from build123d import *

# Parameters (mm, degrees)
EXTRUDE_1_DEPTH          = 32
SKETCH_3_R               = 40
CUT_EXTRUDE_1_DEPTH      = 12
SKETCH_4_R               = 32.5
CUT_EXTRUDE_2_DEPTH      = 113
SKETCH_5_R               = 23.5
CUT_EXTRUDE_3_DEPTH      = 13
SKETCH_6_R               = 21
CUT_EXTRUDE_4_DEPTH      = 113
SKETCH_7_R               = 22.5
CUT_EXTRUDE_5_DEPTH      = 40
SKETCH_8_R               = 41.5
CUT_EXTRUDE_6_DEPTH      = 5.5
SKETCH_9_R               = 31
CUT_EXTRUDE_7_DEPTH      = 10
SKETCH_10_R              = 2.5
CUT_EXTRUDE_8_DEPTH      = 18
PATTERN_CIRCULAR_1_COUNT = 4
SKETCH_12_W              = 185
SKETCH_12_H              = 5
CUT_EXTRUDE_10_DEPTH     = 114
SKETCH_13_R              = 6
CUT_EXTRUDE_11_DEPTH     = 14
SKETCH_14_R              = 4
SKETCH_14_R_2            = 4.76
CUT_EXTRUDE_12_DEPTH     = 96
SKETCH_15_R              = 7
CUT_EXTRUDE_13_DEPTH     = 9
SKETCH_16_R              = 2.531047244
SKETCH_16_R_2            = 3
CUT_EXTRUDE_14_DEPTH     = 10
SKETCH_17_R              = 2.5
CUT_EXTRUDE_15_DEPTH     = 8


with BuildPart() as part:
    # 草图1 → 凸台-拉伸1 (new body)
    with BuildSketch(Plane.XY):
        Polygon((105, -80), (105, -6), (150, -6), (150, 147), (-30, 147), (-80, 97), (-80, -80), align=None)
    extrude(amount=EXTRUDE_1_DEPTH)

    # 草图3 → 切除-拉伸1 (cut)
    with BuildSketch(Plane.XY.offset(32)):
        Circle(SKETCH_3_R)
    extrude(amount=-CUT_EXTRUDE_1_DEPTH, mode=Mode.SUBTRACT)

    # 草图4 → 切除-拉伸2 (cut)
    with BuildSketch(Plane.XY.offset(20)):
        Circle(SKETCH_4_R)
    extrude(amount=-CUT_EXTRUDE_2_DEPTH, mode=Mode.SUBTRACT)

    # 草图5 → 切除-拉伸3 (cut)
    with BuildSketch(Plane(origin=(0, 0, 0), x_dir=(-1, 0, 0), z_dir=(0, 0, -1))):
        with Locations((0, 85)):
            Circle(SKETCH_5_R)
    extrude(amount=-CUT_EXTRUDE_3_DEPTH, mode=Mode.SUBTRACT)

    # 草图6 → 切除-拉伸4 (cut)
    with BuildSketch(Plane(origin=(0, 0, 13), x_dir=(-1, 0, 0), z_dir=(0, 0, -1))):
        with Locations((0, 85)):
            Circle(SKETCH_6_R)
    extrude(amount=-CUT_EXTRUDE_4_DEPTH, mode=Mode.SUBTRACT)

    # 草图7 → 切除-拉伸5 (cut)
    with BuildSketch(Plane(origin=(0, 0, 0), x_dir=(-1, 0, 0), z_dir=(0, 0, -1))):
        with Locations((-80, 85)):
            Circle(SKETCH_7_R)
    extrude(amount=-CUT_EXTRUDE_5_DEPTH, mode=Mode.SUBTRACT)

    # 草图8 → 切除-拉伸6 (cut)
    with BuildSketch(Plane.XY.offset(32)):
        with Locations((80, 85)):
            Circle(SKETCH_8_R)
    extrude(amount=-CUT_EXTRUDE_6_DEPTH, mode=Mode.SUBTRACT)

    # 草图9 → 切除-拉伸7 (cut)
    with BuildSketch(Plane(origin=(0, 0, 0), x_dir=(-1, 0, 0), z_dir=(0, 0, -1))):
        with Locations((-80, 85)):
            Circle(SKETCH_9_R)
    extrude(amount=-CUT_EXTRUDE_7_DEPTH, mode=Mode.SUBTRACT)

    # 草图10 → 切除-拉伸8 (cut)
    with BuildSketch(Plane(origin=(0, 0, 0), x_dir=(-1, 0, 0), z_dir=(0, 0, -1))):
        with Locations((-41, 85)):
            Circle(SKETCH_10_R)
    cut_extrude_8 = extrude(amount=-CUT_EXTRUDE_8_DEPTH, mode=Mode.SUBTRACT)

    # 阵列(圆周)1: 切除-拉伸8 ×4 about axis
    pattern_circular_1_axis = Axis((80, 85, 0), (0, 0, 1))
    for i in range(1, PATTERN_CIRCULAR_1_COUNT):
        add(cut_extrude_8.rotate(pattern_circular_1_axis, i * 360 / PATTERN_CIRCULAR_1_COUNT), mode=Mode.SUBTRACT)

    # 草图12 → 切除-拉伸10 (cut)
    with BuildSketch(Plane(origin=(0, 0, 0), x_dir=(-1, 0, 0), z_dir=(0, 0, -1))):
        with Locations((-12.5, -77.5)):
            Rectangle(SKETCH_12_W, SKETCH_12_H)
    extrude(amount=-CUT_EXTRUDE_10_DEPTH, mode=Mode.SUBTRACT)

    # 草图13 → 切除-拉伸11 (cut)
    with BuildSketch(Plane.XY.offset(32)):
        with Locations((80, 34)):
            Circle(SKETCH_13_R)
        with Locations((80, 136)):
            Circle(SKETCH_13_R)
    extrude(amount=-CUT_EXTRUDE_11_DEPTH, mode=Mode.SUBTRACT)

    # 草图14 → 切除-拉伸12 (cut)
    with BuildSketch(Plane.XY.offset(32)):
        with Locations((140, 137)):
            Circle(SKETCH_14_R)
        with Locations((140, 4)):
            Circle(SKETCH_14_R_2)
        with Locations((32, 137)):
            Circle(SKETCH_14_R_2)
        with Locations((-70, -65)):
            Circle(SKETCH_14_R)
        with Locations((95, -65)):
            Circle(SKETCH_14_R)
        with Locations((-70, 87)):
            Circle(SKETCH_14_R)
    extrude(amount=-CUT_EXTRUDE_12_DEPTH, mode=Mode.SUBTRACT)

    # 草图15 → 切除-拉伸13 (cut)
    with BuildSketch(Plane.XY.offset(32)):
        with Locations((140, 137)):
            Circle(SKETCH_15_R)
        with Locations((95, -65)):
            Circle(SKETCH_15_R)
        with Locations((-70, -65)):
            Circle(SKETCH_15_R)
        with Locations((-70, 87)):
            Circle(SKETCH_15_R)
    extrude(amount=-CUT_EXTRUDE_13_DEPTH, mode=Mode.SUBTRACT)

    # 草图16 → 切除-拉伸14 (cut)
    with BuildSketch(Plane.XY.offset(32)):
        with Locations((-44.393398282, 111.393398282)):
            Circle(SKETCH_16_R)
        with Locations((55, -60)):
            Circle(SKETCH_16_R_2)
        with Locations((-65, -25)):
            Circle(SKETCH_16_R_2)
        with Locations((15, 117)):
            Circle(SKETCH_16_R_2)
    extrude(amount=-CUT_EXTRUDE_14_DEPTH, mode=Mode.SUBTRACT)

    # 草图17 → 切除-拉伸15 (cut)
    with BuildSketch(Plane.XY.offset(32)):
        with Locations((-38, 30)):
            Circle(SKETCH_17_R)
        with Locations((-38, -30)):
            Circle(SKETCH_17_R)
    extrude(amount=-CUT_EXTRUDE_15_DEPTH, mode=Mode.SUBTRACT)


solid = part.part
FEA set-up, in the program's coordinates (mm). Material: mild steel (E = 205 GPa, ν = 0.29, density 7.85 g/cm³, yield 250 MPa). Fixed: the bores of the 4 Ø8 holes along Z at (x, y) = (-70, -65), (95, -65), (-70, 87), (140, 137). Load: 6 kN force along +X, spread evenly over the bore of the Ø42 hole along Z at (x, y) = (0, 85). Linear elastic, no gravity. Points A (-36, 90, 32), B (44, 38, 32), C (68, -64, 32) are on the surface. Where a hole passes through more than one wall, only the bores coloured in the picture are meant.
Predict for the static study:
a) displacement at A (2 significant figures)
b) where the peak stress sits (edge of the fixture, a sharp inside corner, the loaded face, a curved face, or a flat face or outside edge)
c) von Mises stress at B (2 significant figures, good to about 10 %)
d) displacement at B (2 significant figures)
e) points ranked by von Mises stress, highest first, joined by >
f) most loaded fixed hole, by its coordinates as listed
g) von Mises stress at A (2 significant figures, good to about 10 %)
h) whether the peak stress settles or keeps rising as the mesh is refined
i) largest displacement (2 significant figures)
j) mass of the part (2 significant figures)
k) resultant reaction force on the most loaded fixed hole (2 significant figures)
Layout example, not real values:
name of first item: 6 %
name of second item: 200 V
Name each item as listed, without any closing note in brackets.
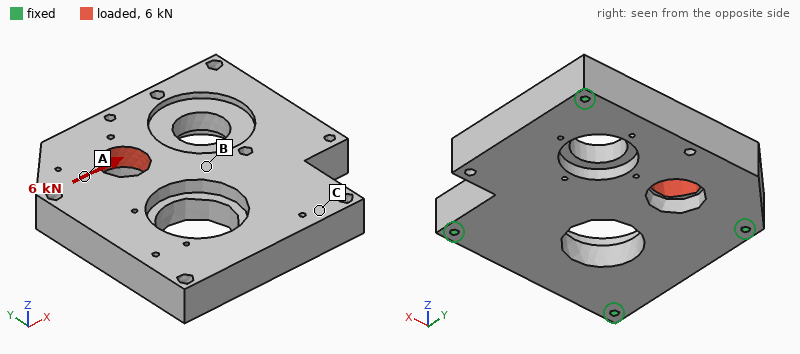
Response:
displacement at A: 0.93 µm
where the peak stress sits: edge of the fixture
von Mises stress at B: 1.1 MPa
displacement at B: 0.99 µm
points ranked by von Mises stress, highest first, joined by >: A > B > C
most loaded fixed hole, by its coordinates as listed: (-70, 87)
von Mises stress at A: 2.9 MPa
whether the peak stress settles or keeps rising as the mesh is refined: keeps rising
largest displacement: 1.6 µm
mass of the part: 9.5 kg
resultant reaction force on the most loaded fixed hole: 3.3 kN
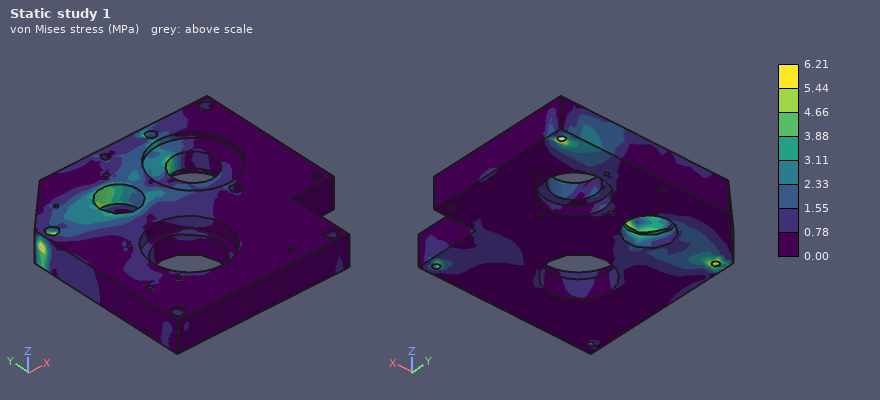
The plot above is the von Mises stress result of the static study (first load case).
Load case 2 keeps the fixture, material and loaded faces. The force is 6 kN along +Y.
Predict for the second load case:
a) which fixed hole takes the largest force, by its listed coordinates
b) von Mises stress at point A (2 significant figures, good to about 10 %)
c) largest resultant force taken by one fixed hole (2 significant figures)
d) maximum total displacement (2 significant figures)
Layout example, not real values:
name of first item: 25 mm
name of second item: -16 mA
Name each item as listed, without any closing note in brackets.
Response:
which fixed hole takes the largest force, by its listed coordinates: (-70, 87)
von Mises stress at point A: 2.0 MPa
largest resultant force taken by one fixed hole: 2.1 kN
maximum total displacement: 2.6 µm
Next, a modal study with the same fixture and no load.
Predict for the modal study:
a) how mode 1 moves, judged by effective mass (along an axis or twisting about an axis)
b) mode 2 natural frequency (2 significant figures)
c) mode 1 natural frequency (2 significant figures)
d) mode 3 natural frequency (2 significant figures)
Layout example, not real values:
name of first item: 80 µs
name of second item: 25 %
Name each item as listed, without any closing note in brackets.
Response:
how mode 1 moves, judged by effective mass: along Z
mode 2 natural frequency: 2500 Hz
mode 1 natural frequency: 2000 Hz
mode 3 natural frequency: 3200 Hz
